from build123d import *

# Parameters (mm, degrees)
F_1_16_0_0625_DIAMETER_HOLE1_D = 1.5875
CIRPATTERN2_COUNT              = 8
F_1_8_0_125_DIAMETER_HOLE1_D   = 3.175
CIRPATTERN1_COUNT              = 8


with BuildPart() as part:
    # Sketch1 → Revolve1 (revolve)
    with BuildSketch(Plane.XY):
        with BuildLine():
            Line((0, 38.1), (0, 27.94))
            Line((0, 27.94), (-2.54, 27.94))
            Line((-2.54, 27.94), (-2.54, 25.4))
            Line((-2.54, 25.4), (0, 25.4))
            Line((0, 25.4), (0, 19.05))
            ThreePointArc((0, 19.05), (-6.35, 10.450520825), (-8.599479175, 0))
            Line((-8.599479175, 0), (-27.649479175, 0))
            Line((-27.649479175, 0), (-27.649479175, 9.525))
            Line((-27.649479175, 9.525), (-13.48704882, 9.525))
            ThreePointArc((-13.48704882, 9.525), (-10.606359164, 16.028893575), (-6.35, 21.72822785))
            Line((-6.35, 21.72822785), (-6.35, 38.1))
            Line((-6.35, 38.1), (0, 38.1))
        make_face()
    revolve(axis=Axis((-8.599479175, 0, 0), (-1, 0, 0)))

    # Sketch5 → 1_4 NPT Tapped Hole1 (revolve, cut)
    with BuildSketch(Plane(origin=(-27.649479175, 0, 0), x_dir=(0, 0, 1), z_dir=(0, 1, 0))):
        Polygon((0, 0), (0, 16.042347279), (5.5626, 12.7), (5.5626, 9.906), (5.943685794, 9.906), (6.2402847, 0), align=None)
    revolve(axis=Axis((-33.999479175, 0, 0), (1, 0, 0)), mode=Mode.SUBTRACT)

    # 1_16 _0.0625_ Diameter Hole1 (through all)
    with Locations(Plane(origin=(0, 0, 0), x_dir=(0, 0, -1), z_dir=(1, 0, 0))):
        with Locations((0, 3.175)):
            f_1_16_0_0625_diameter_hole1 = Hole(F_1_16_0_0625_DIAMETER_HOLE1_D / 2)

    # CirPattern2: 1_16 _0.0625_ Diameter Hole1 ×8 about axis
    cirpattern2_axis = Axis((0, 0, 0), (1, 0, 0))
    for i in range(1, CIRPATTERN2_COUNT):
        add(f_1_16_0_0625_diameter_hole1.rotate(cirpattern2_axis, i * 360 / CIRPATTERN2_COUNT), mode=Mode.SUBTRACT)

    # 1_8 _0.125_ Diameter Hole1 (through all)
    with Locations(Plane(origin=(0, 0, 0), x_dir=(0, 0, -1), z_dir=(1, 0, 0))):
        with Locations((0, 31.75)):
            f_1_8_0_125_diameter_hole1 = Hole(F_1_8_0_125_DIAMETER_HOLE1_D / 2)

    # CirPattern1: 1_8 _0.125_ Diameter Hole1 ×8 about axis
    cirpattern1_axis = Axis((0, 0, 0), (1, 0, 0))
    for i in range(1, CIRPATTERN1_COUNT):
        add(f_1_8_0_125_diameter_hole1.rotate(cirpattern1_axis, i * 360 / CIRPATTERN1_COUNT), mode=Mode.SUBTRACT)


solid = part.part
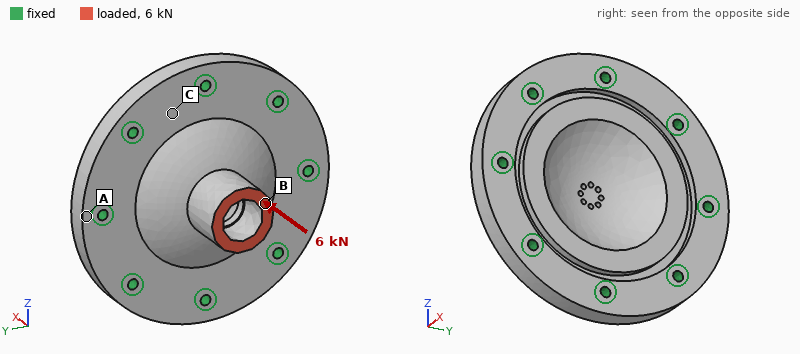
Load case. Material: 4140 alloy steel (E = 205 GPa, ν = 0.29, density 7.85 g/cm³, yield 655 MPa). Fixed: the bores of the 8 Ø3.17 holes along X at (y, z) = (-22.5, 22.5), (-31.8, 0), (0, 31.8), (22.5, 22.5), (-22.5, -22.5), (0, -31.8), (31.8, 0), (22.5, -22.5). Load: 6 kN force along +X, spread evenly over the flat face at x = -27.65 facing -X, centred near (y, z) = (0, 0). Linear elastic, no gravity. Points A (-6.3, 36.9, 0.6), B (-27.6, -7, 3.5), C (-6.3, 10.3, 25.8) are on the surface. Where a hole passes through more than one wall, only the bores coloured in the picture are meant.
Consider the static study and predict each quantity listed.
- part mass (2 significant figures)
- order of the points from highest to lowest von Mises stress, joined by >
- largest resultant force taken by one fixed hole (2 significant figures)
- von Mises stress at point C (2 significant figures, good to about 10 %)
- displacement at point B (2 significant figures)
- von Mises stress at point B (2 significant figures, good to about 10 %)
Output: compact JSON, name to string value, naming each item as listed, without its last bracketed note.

{"part mass": "240 g", "order of the points from highest to lowest von Mises stress, joined by >": "B > C > A", "largest resultant force taken by one fixed hole": "1.2 kN", "von Mises stress at point C": "21 MPa", "displacement at point B": "13 µm", "von Mises stress at point B": "39 MPa"}
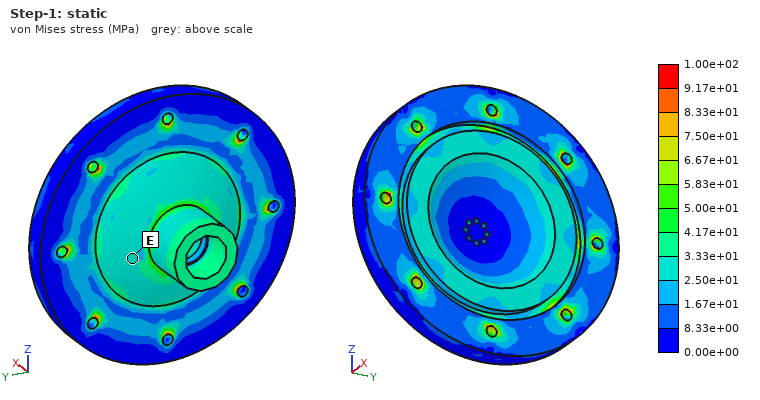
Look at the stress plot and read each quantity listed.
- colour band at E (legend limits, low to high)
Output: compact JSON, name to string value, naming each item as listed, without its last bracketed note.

{"colour band at E": "2.50e+01 to 3.33e+01 MPa"}
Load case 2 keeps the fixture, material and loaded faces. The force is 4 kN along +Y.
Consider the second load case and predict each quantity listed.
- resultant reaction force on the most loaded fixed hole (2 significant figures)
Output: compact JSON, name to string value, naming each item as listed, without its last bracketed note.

{"resultant reaction force on the most loaded fixed hole": "1.3 kN"}
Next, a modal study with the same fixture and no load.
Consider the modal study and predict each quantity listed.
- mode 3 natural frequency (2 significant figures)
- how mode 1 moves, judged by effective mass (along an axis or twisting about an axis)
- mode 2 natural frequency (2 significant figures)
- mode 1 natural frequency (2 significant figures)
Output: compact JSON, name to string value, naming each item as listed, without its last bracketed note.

{"mode 3 natural frequency": "17 kHz", "how mode 1 moves, judged by effective mass": "along X", "mode 2 natural frequency": "17 kHz", "mode 1 natural frequency": "13 kHz"}
